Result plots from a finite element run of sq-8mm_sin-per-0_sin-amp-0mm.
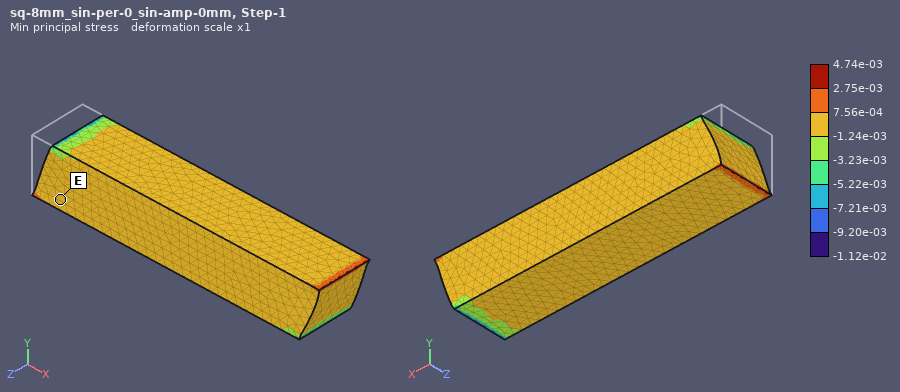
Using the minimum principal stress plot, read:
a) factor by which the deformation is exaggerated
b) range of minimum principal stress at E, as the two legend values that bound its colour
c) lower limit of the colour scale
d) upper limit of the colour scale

1
-1.24e-03 to 7.56e-04
-1.12e-02
4.74e-03
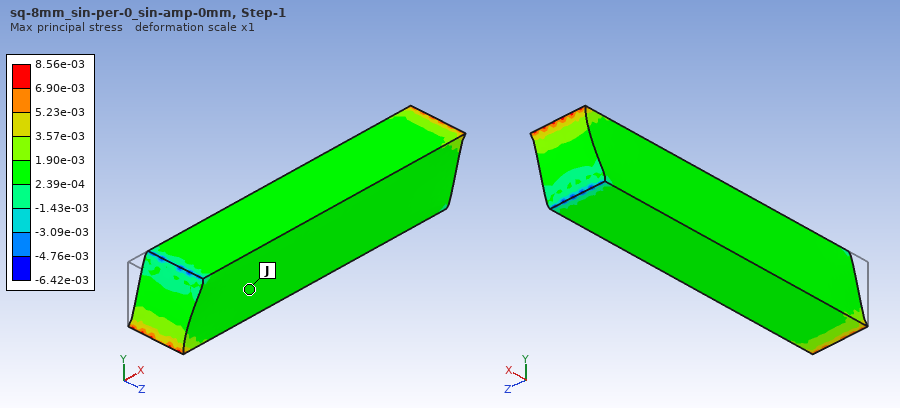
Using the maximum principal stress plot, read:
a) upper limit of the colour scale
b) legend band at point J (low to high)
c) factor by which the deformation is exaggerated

8.56e-03
2.39e-04 to 1.90e-03
1
